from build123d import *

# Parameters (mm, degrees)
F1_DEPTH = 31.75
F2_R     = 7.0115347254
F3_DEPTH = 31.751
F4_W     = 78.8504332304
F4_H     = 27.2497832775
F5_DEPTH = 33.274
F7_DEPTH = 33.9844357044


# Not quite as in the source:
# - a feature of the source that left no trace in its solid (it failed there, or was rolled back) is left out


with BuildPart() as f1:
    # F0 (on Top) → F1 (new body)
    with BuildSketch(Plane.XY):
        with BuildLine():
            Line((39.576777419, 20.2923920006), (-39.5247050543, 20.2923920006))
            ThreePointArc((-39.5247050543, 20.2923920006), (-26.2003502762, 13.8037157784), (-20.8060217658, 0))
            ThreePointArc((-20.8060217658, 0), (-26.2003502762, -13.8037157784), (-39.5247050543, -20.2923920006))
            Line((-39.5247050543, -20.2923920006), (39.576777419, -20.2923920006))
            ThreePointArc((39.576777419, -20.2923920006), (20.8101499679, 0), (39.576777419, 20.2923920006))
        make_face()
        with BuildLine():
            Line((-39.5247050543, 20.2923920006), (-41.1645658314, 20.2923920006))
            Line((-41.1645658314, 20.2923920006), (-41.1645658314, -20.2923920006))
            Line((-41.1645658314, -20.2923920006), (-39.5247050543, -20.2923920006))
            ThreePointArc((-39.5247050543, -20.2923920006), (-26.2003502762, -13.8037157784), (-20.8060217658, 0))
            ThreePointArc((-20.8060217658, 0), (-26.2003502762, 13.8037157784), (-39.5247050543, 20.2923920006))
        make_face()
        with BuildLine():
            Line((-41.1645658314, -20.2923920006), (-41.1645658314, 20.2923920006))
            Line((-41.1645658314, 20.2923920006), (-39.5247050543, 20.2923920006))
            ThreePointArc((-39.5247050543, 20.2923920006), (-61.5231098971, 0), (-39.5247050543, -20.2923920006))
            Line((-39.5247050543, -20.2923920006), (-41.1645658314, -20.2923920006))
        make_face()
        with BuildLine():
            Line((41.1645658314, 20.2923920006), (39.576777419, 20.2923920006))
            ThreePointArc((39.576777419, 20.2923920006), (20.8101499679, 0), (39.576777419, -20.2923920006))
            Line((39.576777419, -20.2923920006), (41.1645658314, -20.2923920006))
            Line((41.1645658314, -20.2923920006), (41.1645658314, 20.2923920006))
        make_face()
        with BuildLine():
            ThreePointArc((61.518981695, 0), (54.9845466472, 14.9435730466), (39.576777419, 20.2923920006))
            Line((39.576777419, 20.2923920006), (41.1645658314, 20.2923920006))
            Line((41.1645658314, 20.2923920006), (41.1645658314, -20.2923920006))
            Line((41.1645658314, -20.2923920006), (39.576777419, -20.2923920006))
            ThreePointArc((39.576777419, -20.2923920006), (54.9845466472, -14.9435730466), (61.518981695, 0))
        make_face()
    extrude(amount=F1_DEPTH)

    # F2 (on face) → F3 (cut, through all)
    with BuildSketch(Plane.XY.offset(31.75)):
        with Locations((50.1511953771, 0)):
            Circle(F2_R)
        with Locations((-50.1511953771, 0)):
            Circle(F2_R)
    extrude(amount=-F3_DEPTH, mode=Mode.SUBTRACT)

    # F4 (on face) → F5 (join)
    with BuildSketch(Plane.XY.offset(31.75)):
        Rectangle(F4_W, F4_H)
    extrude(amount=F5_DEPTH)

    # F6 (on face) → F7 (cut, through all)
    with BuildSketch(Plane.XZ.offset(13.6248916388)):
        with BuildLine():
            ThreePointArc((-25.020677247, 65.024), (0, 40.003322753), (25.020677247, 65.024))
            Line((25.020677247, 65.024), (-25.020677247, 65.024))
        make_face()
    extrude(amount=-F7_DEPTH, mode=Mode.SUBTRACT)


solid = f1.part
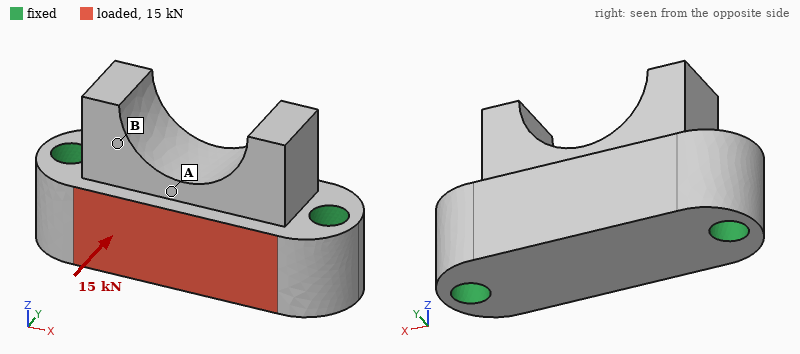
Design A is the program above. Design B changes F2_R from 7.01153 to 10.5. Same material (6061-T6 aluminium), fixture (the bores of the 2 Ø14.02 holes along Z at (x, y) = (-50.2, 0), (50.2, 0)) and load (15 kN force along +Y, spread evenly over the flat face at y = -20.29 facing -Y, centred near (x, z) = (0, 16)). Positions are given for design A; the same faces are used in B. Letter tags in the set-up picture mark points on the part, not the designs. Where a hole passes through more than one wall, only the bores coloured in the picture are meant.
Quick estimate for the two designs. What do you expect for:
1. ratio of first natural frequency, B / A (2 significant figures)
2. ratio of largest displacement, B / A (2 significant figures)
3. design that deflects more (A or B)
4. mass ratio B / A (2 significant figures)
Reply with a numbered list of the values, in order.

1. 1.2
2. 0.76
3. A
4. 0.93
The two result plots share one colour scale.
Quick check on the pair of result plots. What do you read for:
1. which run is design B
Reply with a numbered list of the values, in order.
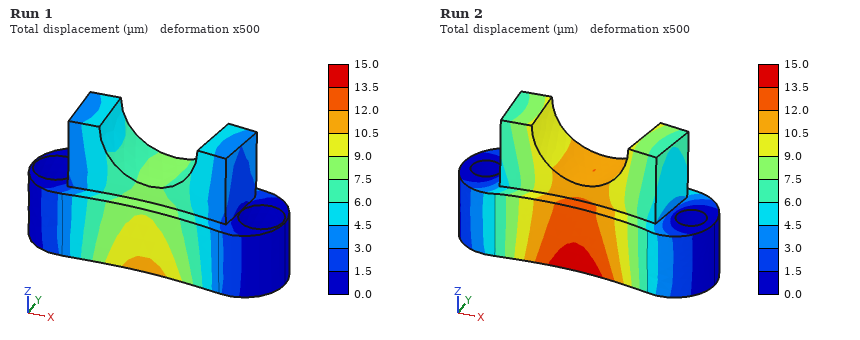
1. Run 1
